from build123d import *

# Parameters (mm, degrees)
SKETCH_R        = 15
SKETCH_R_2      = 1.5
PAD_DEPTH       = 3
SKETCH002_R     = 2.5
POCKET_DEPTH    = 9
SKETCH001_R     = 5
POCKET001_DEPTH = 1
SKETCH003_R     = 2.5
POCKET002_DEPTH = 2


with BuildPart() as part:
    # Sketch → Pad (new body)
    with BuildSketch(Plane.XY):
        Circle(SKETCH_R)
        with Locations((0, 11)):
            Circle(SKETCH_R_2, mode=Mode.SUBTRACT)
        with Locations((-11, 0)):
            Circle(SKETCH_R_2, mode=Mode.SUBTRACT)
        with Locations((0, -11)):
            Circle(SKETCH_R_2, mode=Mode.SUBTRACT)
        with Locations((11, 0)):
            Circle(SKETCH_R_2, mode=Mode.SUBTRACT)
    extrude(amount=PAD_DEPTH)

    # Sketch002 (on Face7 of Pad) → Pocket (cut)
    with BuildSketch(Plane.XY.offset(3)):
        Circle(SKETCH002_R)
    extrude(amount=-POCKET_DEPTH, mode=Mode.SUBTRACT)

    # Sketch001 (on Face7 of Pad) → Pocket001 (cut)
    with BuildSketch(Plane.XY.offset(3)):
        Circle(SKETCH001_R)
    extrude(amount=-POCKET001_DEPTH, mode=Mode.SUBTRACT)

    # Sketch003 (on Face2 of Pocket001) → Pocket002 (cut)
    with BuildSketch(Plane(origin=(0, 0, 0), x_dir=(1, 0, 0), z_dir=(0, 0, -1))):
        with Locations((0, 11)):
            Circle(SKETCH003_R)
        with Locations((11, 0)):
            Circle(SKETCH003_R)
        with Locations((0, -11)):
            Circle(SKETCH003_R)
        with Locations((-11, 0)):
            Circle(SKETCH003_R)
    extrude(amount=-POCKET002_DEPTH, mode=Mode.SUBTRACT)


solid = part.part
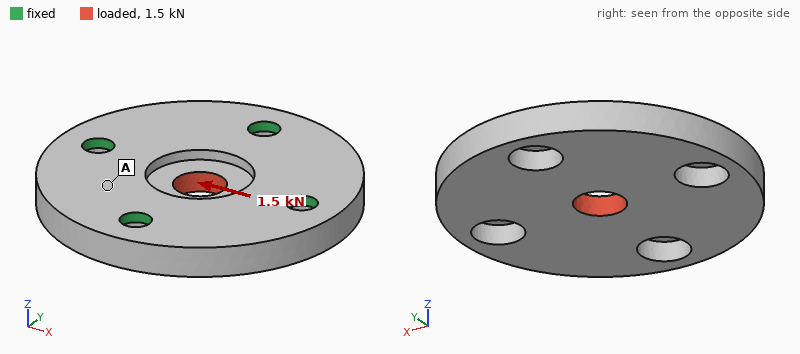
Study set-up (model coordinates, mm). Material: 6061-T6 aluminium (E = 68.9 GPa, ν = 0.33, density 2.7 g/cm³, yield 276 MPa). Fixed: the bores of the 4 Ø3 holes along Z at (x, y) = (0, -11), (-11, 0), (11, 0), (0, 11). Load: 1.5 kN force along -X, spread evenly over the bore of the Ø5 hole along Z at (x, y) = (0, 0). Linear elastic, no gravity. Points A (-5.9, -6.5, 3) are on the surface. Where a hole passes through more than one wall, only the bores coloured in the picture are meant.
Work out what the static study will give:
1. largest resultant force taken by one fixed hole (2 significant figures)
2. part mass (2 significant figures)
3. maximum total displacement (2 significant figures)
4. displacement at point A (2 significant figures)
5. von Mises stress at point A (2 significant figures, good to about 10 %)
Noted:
470 N
4.9 g
6.7 µm
2.2 µm
10 MPa
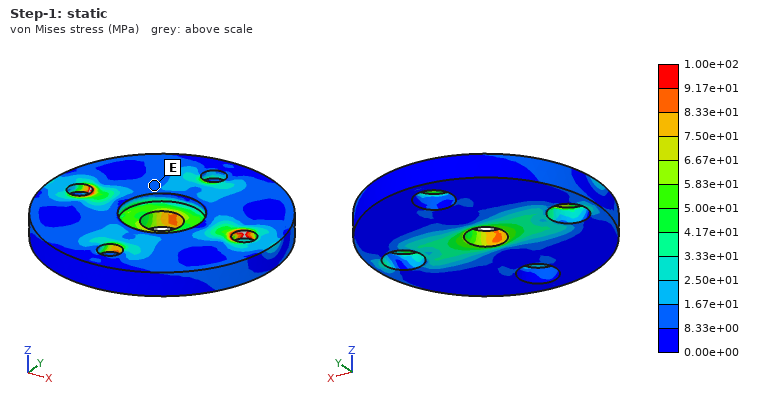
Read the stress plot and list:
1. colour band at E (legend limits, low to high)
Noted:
8.33e+00 to 1.67e+01 MPa
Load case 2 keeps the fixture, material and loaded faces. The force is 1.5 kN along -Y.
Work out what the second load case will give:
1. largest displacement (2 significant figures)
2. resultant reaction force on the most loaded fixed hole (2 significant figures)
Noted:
6.7 µm
470 N
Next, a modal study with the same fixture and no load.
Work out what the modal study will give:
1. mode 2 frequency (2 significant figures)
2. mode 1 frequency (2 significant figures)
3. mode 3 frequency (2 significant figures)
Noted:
29 kHz
26 kHz
29 kHz
